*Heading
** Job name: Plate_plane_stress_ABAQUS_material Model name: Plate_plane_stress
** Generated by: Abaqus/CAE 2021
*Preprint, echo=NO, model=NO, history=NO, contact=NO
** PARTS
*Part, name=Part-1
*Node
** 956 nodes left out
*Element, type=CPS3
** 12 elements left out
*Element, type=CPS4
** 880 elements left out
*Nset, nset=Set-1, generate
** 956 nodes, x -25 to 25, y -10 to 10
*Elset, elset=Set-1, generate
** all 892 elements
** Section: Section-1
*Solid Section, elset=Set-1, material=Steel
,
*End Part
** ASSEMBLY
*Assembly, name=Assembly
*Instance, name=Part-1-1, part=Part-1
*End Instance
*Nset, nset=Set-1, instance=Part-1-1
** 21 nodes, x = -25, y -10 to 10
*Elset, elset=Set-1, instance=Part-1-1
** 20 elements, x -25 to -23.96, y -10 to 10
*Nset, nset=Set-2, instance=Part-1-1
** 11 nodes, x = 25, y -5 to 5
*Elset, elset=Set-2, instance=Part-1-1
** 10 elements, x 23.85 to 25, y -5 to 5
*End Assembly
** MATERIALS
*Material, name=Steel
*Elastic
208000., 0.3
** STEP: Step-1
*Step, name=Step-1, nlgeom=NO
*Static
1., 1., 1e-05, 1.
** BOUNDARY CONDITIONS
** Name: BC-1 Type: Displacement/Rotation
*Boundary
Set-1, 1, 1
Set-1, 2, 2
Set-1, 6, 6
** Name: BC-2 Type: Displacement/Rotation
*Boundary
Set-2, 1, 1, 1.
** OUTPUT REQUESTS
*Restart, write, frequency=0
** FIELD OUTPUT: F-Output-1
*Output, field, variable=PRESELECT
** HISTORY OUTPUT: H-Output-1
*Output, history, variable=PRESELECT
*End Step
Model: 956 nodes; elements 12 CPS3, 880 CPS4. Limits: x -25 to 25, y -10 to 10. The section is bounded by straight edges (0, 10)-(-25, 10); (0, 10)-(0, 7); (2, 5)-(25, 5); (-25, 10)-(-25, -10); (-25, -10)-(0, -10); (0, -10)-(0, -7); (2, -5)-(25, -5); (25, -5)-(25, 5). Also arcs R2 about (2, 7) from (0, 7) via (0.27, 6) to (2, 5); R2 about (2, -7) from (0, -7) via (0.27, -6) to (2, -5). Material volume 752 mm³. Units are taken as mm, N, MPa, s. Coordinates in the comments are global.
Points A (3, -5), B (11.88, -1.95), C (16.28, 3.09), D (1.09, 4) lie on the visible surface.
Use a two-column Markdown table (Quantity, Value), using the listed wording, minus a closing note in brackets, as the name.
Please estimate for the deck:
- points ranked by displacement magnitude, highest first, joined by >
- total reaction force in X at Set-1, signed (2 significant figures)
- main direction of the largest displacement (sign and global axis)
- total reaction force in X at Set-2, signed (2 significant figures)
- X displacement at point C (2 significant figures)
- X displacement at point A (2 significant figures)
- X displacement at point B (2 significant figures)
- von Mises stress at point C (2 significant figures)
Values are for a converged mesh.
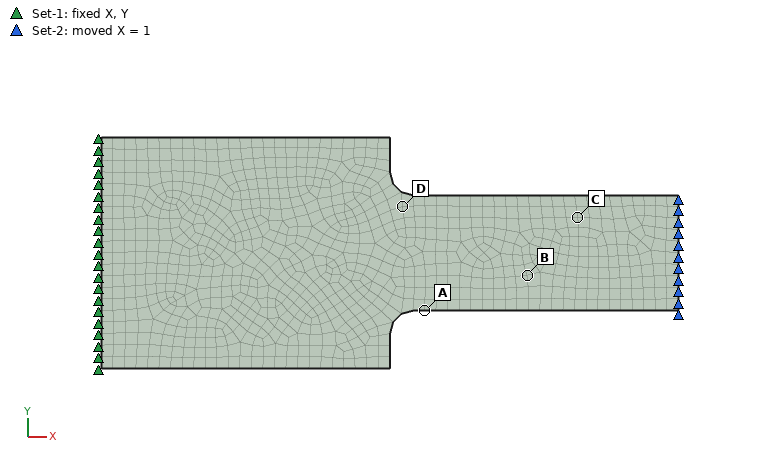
| Quantity | Value |
|---|---|
| points ranked by displacement magnitude, highest first, joined by > | C > B > A > D |
| total reaction force in X at Set-1, signed | -53000 N |
| main direction of the largest displacement | +X |
| total reaction force in X at Set-2, signed | 53000 N |
| X displacement at point C | 0.78 mm |
| X displacement at point A | 0.44 mm |
| X displacement at point B | 0.66 mm |
| von Mises stress at point C | 5300 MPa |
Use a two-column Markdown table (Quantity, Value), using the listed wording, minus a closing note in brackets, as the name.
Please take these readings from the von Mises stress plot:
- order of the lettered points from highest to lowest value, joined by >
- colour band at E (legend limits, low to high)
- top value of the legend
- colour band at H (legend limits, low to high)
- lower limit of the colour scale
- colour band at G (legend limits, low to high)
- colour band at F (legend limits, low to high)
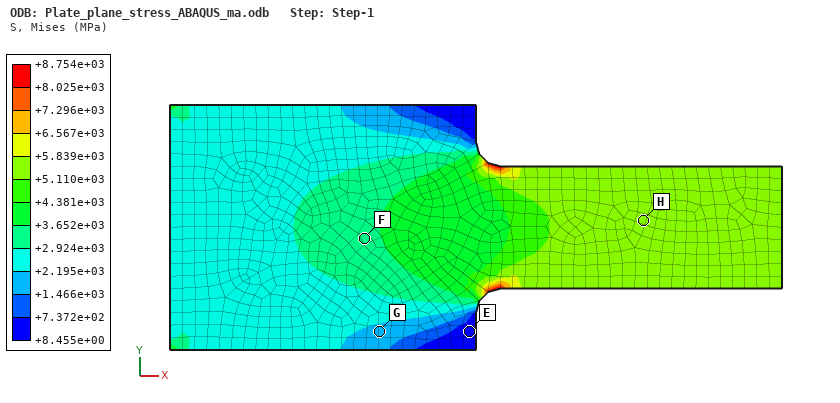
| Quantity | Value |
|---|---|
| order of the lettered points from highest to lowest value, joined by > | H > F > G > E |
| colour band at E | +8.455e+00 to +7.372e+02 MPa |
| top value of the legend | +8.754e+03 MPa |
| colour band at H | +5.110e+03 to +5.839e+03 MPa |
| lower limit of the colour scale | +8.455e+00 MPa |
| colour band at G | +1.466e+03 to +2.195e+03 MPa |
| colour band at F | +2.924e+03 to +3.652e+03 MPa |
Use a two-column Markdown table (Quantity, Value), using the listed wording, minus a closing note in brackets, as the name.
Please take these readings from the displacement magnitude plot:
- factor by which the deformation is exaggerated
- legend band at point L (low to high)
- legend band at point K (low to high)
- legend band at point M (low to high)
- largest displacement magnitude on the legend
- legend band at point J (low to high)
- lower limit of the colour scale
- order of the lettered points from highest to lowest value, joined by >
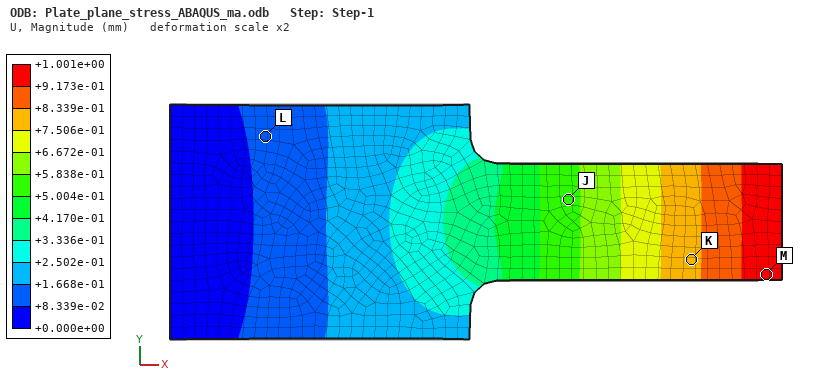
| Quantity | Value |
|---|---|
| factor by which the deformation is exaggerated | 2 |
| legend band at point L | +8.339e-02 to +1.668e-01 mm |
| legend band at point K | +7.506e-01 to +8.339e-01 mm |
| legend band at point M | +9.173e-01 to +1.001e+00 mm |
| largest displacement magnitude on the legend | +1.001e+00 mm |
| legend band at point J | +5.004e-01 to +5.838e-01 mm |
| lower limit of the colour scale | +0.000e+00 mm |
| order of the lettered points from highest to lowest value, joined by > | M > K > J > L |
